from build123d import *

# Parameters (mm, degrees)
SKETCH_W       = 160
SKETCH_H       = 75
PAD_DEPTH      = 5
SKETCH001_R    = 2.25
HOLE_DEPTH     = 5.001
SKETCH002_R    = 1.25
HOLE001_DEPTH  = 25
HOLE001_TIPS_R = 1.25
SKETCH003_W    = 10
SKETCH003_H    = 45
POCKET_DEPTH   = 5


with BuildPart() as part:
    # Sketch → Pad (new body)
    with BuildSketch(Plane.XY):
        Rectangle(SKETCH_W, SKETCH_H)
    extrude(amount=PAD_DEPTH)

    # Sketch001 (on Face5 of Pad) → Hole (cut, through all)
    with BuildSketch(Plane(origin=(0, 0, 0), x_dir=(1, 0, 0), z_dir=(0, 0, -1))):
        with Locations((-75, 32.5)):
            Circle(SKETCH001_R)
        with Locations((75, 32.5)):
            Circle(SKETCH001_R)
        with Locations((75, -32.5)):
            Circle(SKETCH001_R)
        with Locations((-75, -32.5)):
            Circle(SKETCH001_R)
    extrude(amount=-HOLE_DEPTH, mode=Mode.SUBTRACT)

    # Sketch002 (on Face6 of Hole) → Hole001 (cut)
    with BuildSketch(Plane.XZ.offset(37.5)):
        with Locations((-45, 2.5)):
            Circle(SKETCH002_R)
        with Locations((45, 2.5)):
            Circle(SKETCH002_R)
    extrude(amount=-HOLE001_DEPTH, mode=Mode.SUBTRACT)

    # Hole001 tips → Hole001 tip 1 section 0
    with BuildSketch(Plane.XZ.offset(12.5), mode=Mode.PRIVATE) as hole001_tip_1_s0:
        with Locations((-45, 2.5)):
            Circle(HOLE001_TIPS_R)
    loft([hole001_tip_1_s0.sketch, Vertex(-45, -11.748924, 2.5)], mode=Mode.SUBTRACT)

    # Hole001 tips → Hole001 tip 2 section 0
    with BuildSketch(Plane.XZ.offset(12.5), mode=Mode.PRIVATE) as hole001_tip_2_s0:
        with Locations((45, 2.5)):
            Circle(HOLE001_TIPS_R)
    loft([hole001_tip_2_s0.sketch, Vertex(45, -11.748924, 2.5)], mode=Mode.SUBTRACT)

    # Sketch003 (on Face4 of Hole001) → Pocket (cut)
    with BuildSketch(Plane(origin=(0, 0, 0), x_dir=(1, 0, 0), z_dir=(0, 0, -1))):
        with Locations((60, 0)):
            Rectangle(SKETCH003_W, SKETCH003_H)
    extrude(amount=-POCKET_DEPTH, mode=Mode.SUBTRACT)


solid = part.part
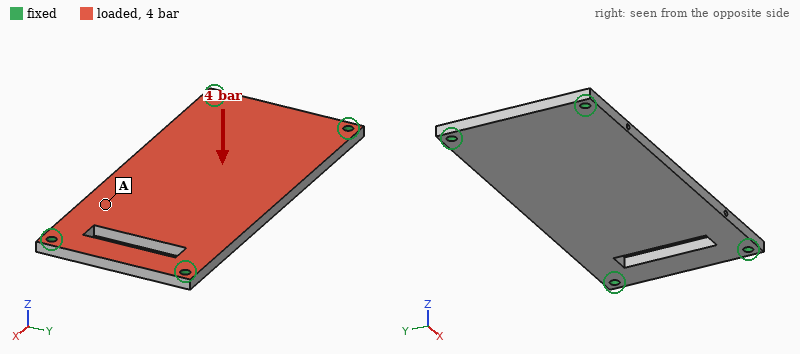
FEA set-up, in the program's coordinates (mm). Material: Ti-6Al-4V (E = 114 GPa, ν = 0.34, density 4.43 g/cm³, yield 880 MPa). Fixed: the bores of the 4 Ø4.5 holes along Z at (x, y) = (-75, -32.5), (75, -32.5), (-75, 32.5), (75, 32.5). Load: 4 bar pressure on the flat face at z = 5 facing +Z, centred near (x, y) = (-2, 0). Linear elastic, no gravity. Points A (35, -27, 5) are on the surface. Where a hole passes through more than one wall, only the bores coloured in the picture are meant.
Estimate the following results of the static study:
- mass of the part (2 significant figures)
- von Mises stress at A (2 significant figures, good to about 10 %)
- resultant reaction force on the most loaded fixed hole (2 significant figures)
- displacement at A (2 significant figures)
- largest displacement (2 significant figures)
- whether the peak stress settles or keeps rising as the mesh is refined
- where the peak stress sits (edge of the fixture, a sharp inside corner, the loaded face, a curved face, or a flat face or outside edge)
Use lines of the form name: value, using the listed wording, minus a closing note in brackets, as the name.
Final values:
mass of the part: 250 g
von Mises stress at A: 65 MPa
resultant reaction force on the most loaded fixed hole: 1.2 kN
displacement at A: 0.42 mm
largest displacement: 0.66 mm
whether the peak stress settles or keeps rising as the mesh is refined: keeps rising
where the peak stress sits: edge of the fixture
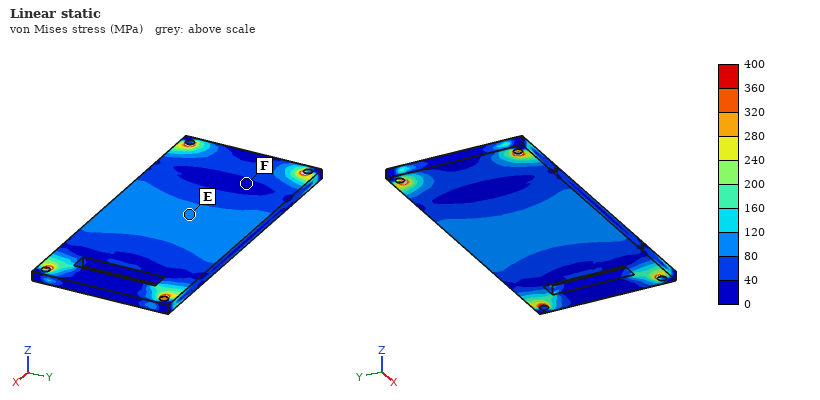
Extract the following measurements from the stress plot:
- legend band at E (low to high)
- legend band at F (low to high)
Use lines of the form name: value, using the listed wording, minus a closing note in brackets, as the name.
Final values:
legend band at E: 80 to 120 MPa
legend band at F: 0 to 40 MPa
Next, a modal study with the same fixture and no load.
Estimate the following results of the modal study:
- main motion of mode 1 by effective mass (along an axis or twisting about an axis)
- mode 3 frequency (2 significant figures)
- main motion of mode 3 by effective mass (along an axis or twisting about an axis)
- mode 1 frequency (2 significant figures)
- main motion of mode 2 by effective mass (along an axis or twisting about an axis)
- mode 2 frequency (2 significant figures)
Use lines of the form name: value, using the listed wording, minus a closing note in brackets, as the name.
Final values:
main motion of mode 1 by effective mass: along Z
mode 3 frequency: 2700 Hz
main motion of mode 3 by effective mass: twisting about Y
mode 1 frequency: 960 Hz
main motion of mode 2 by effective mass: twisting about X
mode 2 frequency: 1800 Hz
